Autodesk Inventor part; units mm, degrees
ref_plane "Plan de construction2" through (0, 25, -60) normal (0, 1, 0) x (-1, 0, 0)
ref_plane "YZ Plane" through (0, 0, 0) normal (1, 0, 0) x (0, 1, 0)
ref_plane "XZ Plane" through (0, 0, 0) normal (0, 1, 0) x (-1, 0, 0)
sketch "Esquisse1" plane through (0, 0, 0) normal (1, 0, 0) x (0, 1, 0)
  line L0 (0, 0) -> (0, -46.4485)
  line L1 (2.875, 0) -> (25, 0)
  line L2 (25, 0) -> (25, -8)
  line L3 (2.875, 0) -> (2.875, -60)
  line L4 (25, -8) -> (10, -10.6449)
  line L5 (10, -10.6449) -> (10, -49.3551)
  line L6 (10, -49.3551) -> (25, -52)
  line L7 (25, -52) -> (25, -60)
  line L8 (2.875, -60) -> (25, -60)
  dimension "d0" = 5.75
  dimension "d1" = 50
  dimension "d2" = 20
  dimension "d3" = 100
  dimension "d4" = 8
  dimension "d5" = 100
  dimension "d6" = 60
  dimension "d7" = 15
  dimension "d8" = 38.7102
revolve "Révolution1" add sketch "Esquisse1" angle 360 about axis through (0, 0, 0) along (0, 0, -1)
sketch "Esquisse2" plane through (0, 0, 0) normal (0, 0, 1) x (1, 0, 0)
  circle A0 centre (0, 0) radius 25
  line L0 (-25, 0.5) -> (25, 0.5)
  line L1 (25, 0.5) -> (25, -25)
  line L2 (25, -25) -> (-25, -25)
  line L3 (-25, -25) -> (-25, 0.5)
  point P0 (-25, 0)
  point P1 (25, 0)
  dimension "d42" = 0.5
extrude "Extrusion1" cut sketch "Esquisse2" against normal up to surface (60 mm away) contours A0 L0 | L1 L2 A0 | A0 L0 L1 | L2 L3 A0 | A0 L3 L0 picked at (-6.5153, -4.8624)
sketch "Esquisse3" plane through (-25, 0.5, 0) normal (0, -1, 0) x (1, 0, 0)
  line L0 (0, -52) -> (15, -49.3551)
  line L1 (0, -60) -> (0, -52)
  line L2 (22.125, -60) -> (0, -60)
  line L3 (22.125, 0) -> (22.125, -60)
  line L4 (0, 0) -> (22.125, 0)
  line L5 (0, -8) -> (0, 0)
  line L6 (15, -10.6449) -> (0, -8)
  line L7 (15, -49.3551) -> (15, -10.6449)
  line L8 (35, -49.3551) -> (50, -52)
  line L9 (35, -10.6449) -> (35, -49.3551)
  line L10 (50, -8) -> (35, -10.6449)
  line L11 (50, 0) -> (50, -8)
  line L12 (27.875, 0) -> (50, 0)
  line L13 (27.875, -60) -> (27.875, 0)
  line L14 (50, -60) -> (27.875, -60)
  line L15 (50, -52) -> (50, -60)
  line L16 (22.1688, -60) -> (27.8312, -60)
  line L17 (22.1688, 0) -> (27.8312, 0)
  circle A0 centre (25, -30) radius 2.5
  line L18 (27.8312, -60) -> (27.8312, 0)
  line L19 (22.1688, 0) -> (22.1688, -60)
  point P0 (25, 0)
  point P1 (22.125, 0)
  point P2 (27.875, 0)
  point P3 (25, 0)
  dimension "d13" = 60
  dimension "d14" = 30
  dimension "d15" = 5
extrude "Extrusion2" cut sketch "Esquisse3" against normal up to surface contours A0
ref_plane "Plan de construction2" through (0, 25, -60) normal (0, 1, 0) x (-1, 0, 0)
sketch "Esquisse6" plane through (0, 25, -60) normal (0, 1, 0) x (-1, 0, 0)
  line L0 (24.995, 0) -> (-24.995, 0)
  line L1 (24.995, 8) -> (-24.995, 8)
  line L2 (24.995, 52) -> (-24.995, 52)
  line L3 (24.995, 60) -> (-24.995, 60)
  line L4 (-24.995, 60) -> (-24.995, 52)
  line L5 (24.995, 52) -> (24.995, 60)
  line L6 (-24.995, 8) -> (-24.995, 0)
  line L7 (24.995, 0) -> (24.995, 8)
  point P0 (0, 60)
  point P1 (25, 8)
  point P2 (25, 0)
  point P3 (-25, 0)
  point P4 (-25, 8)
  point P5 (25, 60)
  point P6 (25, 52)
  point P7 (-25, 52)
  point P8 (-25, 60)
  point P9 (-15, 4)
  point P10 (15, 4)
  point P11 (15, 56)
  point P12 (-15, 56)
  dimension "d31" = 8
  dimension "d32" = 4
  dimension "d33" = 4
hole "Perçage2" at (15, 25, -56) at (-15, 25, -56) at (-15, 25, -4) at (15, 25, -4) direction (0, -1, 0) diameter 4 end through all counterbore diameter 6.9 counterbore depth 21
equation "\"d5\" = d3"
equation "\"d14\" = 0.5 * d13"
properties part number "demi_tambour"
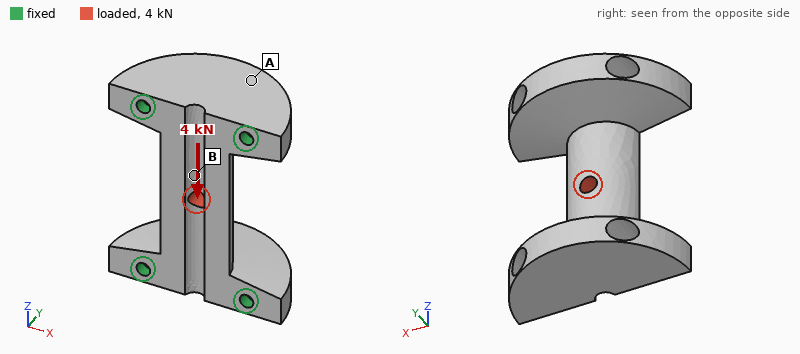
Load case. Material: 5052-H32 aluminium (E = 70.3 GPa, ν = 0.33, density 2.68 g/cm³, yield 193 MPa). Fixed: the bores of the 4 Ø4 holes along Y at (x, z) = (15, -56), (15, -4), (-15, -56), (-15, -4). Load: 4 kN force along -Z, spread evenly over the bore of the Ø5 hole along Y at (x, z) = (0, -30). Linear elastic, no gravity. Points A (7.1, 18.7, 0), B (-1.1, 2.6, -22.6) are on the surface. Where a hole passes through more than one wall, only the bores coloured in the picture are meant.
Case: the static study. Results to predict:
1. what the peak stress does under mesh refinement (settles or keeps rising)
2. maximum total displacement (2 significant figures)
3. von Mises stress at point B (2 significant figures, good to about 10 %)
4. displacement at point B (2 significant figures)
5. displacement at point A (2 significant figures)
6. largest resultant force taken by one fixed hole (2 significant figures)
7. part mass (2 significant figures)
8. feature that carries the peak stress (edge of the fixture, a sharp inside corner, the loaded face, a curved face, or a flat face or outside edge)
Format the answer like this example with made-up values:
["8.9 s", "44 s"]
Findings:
["keeps rising", "13 µm", "24 MPa", "11 µm", "10 µm", "1.1 kN", "54 g", "edge of the fixture"]
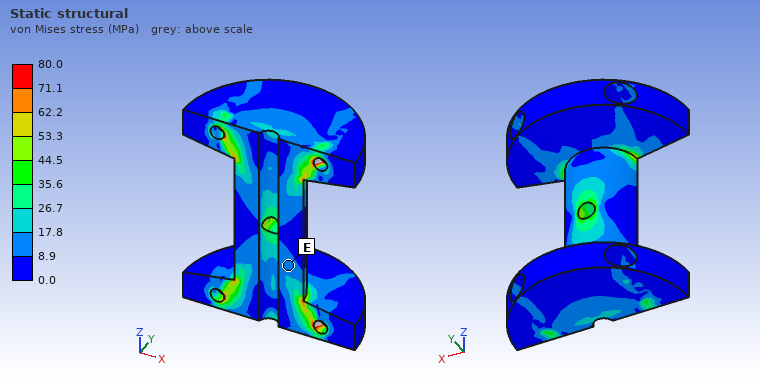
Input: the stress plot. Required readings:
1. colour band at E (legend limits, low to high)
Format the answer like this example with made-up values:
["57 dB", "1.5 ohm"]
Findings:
["8.9 to 17.8 MPa"]
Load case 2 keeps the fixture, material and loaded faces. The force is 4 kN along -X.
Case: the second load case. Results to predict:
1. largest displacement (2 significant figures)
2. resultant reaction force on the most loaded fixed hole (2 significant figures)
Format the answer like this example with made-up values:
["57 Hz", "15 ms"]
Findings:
["30 µm", "1.4 kN"]
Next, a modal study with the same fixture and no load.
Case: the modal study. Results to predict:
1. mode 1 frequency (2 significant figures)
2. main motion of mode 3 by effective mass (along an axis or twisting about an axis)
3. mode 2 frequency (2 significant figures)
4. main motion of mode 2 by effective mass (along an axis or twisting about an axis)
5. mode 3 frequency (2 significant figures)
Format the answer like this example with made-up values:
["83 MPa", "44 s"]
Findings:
["7600 Hz", "along Y", "11 kHz", "along Z", "18 kHz"]
